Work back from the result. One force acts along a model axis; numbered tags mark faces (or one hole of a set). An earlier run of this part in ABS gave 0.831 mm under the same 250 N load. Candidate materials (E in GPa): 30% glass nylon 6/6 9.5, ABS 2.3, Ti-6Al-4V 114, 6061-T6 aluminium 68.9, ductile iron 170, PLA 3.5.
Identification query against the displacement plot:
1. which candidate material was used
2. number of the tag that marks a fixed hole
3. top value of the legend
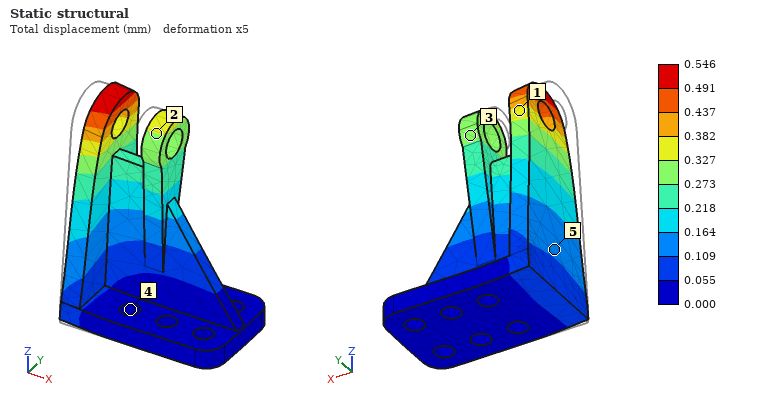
PLA
4
0.546 mm
